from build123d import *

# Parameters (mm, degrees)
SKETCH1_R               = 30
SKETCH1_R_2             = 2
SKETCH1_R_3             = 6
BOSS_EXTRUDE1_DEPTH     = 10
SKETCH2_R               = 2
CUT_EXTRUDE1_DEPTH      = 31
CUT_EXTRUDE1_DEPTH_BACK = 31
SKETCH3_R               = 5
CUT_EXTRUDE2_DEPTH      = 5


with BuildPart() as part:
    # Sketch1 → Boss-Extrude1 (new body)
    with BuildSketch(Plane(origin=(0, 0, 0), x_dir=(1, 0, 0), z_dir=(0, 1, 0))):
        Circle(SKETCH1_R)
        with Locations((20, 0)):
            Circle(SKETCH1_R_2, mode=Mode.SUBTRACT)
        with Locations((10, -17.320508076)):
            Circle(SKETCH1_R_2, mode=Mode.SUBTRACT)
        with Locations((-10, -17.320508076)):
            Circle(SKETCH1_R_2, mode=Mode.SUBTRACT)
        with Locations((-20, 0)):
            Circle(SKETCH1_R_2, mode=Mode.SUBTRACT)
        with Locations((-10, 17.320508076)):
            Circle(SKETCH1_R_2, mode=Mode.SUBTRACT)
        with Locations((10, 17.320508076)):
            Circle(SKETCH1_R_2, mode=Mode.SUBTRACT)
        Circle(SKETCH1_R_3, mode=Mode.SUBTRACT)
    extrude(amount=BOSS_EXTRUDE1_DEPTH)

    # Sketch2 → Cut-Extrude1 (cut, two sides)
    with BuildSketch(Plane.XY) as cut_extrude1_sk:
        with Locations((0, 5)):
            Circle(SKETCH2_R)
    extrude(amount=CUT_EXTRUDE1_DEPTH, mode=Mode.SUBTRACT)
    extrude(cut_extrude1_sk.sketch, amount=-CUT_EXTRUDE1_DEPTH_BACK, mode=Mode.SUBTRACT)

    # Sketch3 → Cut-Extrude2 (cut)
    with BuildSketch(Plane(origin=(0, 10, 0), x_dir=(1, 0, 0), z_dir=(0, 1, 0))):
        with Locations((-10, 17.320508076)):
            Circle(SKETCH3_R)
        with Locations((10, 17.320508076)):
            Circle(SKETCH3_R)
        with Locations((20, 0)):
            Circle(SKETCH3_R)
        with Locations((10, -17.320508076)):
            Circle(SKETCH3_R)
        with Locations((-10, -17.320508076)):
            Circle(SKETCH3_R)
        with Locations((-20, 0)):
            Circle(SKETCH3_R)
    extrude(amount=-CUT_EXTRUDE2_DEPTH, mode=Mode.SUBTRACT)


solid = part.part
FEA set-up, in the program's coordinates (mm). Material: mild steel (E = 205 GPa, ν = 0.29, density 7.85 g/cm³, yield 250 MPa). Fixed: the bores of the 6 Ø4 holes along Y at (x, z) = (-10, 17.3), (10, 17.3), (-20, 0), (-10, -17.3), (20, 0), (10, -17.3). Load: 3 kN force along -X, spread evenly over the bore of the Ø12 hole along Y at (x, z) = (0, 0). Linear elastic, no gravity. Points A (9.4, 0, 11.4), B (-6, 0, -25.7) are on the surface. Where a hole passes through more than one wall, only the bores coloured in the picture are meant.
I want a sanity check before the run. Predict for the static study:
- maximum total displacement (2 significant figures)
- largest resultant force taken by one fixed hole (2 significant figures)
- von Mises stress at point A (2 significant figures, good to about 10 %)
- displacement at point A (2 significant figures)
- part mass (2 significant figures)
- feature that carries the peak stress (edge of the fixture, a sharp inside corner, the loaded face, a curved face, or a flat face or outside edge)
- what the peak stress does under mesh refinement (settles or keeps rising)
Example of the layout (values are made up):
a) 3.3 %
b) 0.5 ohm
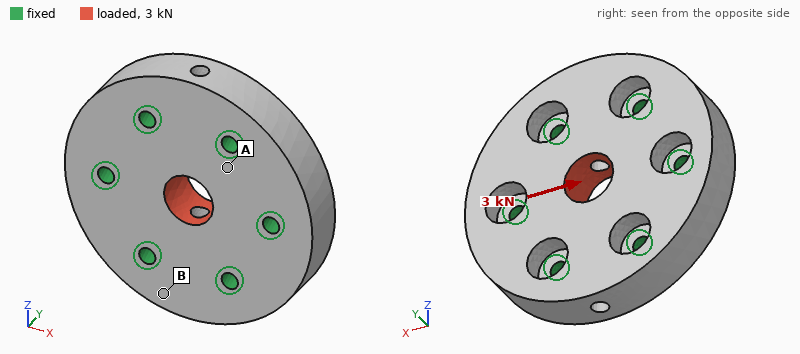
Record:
a) 0.88 µm
b) 720 N
c) 4.0 MPa
d) 0.23 µm
e) 190 g
f) edge of the fixture
g) keeps rising
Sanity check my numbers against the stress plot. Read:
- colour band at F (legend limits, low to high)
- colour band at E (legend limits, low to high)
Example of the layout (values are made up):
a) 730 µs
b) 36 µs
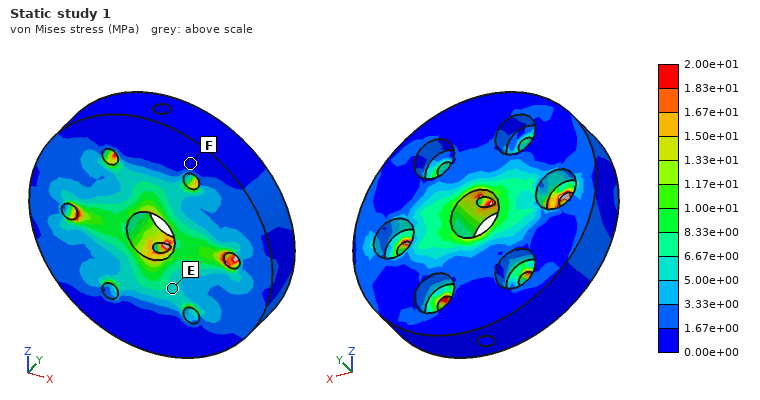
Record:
a) 0.00e+00 to 1.67e+00 MPa
b) 5.00e+00 to 6.67e+00 MPa
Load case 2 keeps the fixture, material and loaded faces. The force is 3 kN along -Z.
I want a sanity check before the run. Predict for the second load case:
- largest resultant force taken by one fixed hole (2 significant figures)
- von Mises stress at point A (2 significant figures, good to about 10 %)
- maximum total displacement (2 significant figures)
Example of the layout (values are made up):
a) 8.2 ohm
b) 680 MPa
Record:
a) 620 N
b) 8.5 MPa
c) 0.81 µm
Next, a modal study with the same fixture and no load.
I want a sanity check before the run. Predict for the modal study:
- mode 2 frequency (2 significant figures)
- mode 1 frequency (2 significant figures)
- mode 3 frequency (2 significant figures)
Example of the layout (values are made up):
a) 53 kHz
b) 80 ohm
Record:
a) 26 kHz
b) 25 kHz
c) 26 kHz
